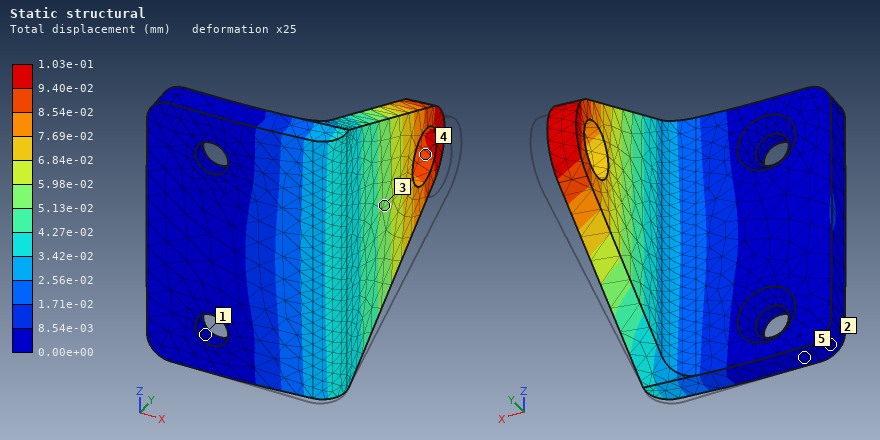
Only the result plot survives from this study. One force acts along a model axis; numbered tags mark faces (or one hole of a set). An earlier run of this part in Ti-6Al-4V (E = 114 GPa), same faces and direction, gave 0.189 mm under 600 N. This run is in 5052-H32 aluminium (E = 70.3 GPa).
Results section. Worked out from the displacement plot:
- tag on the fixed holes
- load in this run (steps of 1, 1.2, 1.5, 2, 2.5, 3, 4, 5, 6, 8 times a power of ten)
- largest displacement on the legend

1
200 N
1.03e-01 mm
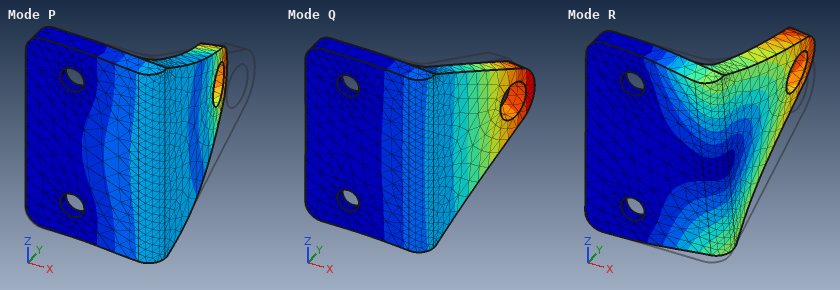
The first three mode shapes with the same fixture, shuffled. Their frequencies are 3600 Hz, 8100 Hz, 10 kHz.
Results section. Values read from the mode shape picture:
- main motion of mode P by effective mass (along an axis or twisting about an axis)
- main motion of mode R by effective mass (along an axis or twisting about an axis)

along Y
along Z
